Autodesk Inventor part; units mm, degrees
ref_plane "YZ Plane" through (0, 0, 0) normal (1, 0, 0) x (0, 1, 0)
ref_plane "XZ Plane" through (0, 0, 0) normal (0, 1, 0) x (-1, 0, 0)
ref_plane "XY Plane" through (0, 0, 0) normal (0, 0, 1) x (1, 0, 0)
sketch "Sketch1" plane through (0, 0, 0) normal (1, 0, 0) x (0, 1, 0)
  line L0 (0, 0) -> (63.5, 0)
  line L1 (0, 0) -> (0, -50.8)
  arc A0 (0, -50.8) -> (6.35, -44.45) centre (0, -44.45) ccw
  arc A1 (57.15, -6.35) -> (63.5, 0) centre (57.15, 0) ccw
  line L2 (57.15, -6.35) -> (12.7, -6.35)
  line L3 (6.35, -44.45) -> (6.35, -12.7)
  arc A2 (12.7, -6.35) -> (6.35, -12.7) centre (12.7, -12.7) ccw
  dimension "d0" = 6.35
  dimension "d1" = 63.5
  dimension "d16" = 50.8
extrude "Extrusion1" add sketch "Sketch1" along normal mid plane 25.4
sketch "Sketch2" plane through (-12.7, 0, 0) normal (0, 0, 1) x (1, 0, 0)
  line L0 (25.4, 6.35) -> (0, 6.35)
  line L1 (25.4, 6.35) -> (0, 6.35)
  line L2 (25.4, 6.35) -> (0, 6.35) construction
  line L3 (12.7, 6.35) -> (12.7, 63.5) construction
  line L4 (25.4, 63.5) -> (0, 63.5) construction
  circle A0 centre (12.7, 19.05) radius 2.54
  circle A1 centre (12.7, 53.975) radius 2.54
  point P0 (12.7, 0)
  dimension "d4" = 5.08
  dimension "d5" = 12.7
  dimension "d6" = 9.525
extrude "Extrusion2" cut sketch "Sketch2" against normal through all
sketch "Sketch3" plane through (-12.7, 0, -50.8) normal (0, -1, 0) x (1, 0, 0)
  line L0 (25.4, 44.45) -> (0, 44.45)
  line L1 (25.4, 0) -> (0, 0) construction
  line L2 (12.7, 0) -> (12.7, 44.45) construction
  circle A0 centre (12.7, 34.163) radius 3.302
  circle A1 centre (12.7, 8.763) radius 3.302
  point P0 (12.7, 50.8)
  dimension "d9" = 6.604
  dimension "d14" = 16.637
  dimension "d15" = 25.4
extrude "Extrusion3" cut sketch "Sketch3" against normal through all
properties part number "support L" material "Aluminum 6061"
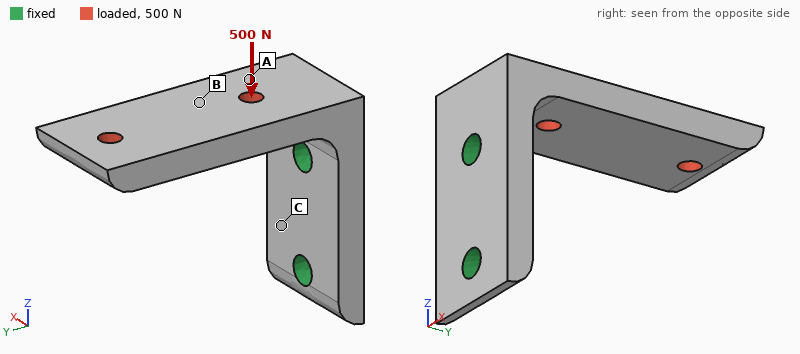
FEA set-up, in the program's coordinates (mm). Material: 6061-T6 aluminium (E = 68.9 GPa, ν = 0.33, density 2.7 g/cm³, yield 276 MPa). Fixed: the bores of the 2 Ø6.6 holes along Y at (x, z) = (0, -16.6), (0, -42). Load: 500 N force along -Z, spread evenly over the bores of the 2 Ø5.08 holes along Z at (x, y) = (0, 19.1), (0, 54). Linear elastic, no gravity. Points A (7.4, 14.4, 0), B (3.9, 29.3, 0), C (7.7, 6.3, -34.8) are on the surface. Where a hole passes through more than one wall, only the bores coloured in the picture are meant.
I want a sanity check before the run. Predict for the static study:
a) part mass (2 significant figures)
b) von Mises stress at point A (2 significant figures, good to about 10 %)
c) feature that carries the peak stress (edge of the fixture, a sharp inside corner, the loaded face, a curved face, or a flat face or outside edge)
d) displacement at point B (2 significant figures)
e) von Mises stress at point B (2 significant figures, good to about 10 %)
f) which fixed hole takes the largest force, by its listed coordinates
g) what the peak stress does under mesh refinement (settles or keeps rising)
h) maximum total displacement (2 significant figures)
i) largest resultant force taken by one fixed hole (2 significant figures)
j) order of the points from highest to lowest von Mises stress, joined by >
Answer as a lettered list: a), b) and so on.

a) 45 g
b) 67 MPa
c) edge of the fixture
d) 0.18 mm
e) 36 MPa
f) (0, -16.6)
g) keeps rising
h) 0.57 mm
i) 490 N
j) A > B > C
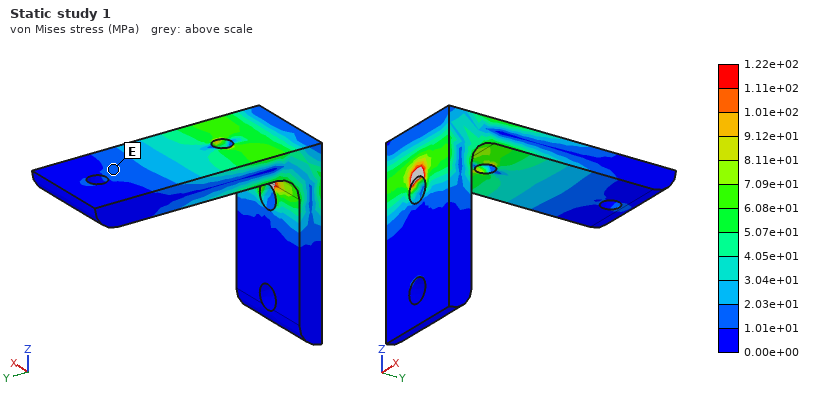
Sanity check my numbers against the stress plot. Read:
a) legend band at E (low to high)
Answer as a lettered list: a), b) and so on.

a) 1.01e+01 to 2.03e+01 MPa
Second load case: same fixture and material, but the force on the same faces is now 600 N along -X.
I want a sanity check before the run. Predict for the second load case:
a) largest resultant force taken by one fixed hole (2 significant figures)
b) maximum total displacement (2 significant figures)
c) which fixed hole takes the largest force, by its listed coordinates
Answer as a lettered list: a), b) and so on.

a) 770 N
b) 0.21 mm
c) (0, -16.6)
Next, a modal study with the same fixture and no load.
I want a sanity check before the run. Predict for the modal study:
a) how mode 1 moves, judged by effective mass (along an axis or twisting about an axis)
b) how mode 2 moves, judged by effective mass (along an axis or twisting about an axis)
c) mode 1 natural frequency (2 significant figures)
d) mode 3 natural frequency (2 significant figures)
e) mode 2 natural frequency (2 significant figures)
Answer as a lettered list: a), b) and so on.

a) along Z
b) along X
c) 1300 Hz
d) 6300 Hz
e) 2200 Hz
